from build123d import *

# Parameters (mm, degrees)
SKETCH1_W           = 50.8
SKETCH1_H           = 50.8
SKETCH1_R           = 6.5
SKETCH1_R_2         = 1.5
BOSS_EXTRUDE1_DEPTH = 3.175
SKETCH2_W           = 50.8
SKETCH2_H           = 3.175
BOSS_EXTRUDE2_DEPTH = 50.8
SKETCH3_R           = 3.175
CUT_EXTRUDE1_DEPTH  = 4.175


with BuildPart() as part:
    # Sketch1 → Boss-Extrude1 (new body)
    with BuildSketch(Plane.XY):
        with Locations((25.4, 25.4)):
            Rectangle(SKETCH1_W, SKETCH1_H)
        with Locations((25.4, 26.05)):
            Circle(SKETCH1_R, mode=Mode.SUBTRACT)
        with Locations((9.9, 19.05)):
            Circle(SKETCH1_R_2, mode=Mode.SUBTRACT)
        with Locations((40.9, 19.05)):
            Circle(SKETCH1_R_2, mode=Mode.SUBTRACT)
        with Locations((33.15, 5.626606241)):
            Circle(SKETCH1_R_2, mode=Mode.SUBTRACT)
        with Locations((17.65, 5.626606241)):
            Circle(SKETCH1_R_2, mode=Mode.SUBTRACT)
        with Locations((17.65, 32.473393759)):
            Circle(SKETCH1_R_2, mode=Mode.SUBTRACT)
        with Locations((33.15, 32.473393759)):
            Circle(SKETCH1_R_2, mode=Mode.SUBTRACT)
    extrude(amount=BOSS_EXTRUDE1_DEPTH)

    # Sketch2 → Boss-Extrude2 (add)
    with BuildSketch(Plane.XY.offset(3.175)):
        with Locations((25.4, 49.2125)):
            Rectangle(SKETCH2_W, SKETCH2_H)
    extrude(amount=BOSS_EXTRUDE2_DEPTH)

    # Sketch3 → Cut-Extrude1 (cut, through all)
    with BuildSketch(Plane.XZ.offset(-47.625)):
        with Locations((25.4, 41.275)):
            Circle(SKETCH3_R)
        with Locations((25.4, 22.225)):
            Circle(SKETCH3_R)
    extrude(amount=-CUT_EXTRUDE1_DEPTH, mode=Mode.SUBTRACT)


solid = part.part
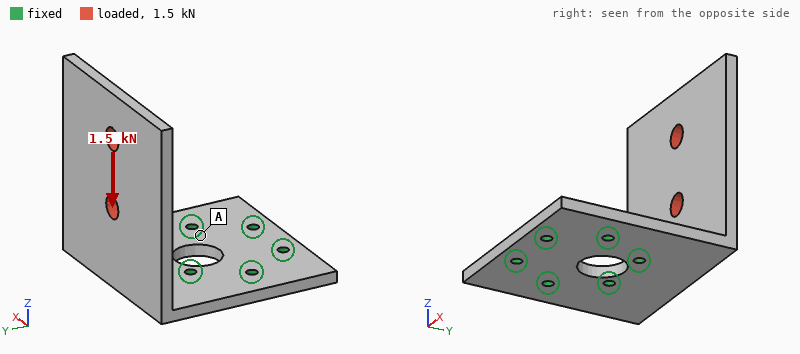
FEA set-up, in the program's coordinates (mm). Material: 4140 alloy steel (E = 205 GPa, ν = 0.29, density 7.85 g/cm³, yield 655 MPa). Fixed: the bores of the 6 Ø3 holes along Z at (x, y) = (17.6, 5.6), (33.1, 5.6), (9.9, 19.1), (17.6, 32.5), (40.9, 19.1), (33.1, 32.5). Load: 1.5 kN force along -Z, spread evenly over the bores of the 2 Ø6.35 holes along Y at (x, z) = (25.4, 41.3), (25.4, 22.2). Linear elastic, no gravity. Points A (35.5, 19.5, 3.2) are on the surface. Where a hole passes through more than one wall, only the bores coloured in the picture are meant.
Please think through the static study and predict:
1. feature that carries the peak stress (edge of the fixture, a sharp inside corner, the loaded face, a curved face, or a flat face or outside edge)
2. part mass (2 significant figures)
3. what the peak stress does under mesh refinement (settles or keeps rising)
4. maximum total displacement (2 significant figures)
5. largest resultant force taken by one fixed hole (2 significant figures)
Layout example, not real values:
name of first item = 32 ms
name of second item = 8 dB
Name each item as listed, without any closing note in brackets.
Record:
feature that carries the peak stress = edge of the fixture
part mass = 120 g
what the peak stress does under mesh refinement = keeps rising
maximum total displacement = 0.46 mm
largest resultant force taken by one fixed hole = 1.0 kN
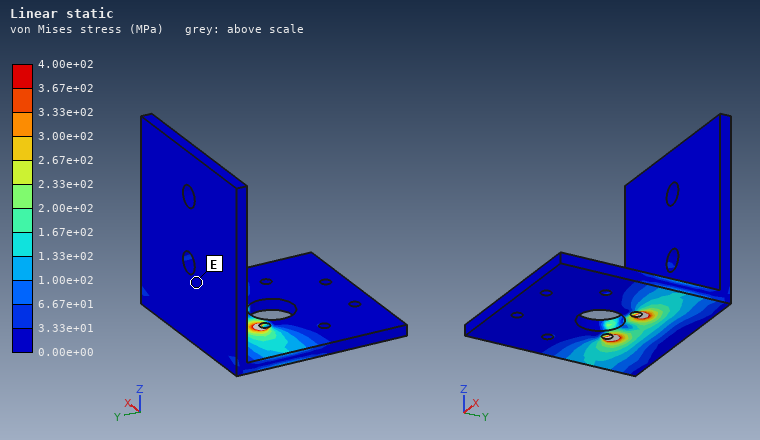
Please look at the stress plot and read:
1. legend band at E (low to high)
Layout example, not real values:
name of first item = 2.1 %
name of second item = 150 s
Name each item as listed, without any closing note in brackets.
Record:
legend band at E = 0.00e+00 to 3.33e+01 MPa
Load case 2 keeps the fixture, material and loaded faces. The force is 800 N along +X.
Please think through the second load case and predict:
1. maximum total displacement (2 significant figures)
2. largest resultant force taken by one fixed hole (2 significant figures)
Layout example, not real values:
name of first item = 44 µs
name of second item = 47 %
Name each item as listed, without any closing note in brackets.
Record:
maximum total displacement = 0.28 mm
largest resultant force taken by one fixed hole = 1.1 kN
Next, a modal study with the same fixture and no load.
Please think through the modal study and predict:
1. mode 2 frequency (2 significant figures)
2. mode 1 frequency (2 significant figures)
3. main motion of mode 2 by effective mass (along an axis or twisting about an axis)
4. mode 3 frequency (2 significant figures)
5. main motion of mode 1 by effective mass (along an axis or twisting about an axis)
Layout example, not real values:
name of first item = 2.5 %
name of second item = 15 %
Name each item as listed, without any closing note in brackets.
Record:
mode 2 frequency = 1300 Hz
mode 1 frequency = 640 Hz
main motion of mode 2 by effective mass = along X
mode 3 frequency = 2300 Hz
main motion of mode 1 by effective mass = along Y
